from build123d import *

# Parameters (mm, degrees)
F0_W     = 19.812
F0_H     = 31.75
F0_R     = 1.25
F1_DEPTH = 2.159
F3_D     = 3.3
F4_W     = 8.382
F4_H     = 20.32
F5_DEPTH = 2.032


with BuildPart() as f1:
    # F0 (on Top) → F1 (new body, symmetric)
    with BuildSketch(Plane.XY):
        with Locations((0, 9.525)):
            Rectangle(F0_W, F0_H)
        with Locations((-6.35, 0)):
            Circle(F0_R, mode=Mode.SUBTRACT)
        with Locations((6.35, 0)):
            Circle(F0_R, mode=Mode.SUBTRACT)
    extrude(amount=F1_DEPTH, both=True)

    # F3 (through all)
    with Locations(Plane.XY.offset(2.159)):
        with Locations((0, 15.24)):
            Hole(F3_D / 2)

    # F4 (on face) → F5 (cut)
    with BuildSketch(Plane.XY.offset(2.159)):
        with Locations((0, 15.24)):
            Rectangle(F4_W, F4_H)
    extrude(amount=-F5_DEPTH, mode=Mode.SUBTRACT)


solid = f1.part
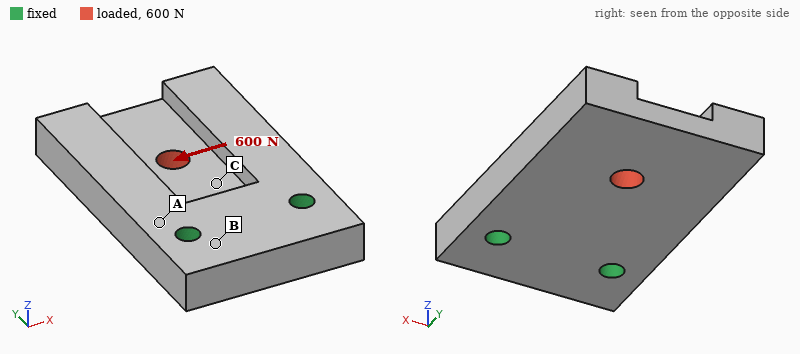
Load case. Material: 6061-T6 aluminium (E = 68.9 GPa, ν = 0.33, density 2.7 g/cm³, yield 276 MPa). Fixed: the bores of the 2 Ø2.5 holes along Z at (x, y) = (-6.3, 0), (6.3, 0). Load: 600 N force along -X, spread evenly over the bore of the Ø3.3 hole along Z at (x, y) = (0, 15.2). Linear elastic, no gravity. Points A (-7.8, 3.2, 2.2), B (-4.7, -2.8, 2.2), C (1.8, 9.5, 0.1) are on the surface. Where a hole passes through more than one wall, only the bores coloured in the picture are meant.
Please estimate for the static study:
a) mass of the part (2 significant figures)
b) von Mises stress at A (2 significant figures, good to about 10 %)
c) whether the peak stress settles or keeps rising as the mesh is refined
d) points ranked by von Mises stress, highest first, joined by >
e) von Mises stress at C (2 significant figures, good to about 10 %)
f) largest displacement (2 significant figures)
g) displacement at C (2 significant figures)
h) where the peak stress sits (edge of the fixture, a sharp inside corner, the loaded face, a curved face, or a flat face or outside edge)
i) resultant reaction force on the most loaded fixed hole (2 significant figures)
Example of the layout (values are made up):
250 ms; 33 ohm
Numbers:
6.2 g; 20 MPa; keeps rising; C > A > B; 33 MPa; 18 µm; 6.2 µm; edge of the fixture; 700 N
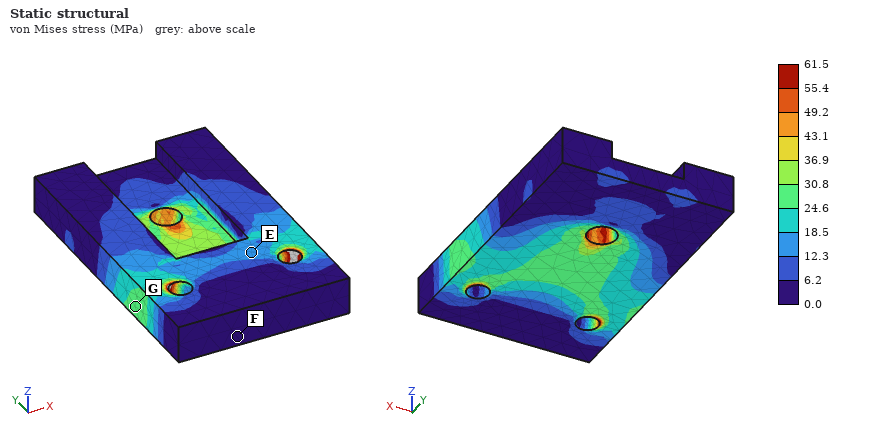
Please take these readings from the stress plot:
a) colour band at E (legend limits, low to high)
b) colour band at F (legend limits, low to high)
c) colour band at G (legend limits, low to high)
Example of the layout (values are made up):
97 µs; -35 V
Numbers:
12.3 to 18.5 MPa; 0.0 to 6.2 MPa; 24.6 to 30.8 MPa
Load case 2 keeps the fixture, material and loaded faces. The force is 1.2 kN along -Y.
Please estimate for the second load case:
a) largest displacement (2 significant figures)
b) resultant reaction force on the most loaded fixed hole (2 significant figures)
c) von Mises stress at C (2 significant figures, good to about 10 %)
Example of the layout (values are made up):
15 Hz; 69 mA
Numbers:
36 µm; 610 N; 28 MPa
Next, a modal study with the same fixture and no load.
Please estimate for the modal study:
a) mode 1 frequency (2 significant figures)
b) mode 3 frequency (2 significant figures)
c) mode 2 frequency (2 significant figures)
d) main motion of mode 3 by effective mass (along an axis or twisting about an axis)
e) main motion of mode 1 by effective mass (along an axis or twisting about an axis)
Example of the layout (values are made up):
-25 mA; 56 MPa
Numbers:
5400 Hz; 18 kHz; 11 kHz; along X; along Z
